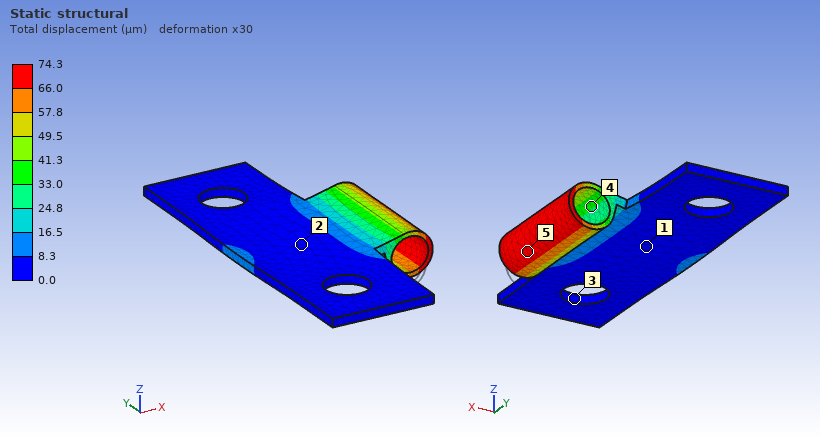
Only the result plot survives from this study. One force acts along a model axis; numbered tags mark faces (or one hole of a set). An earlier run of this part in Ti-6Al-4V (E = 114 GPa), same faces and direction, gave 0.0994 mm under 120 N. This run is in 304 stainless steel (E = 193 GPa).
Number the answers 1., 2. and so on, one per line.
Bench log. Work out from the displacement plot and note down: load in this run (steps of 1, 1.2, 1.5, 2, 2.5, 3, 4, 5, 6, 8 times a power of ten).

1. 150 N
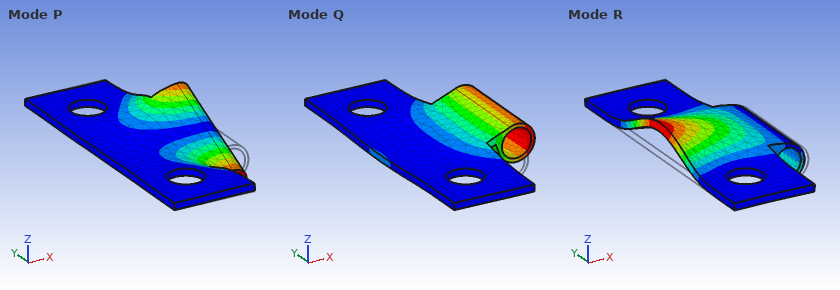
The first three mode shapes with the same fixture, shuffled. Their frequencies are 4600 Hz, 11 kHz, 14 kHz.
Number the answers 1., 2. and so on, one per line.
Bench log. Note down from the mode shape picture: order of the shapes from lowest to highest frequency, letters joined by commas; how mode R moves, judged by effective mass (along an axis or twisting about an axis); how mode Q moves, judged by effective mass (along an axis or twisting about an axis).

1. Q, R, P
2. along Z
3. along Z
